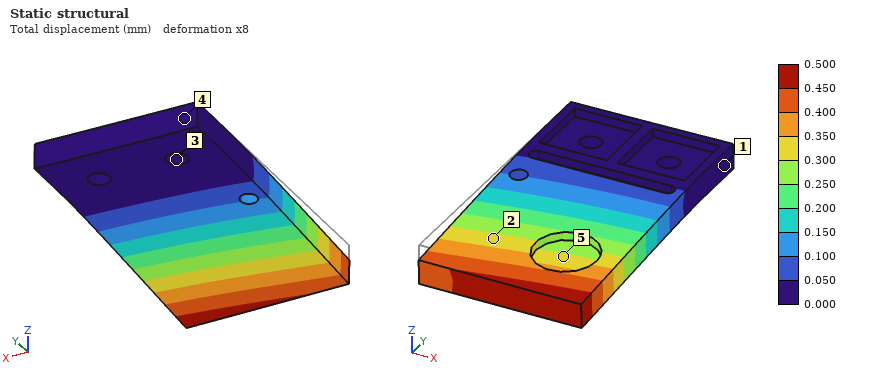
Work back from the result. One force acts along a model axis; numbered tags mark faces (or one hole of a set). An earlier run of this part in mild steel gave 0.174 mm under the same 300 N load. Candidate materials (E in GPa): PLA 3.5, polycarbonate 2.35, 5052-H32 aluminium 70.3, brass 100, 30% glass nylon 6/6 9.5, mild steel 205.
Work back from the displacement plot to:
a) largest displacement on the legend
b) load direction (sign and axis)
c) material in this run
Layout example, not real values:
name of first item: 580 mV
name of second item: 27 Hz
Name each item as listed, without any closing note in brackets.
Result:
largest displacement on the legend: 0.500 mm
load direction: -Z
material in this run: 5052-H32 aluminium
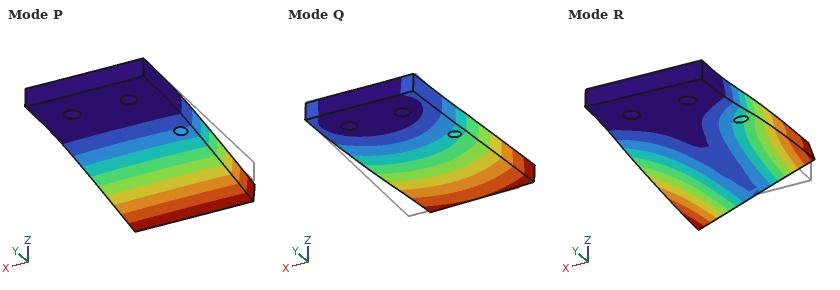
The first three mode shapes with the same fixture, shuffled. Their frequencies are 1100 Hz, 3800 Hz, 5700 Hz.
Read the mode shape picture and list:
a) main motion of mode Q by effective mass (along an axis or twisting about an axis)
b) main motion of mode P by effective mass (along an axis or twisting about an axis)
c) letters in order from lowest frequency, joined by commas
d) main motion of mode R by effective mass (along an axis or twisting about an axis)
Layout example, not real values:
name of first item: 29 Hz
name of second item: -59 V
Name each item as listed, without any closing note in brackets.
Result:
main motion of mode Q by effective mass: along X
main motion of mode P by effective mass: along Z
letters in order from lowest frequency, joined by commas: P, R, Q
main motion of mode R by effective mass: twisting about Y
